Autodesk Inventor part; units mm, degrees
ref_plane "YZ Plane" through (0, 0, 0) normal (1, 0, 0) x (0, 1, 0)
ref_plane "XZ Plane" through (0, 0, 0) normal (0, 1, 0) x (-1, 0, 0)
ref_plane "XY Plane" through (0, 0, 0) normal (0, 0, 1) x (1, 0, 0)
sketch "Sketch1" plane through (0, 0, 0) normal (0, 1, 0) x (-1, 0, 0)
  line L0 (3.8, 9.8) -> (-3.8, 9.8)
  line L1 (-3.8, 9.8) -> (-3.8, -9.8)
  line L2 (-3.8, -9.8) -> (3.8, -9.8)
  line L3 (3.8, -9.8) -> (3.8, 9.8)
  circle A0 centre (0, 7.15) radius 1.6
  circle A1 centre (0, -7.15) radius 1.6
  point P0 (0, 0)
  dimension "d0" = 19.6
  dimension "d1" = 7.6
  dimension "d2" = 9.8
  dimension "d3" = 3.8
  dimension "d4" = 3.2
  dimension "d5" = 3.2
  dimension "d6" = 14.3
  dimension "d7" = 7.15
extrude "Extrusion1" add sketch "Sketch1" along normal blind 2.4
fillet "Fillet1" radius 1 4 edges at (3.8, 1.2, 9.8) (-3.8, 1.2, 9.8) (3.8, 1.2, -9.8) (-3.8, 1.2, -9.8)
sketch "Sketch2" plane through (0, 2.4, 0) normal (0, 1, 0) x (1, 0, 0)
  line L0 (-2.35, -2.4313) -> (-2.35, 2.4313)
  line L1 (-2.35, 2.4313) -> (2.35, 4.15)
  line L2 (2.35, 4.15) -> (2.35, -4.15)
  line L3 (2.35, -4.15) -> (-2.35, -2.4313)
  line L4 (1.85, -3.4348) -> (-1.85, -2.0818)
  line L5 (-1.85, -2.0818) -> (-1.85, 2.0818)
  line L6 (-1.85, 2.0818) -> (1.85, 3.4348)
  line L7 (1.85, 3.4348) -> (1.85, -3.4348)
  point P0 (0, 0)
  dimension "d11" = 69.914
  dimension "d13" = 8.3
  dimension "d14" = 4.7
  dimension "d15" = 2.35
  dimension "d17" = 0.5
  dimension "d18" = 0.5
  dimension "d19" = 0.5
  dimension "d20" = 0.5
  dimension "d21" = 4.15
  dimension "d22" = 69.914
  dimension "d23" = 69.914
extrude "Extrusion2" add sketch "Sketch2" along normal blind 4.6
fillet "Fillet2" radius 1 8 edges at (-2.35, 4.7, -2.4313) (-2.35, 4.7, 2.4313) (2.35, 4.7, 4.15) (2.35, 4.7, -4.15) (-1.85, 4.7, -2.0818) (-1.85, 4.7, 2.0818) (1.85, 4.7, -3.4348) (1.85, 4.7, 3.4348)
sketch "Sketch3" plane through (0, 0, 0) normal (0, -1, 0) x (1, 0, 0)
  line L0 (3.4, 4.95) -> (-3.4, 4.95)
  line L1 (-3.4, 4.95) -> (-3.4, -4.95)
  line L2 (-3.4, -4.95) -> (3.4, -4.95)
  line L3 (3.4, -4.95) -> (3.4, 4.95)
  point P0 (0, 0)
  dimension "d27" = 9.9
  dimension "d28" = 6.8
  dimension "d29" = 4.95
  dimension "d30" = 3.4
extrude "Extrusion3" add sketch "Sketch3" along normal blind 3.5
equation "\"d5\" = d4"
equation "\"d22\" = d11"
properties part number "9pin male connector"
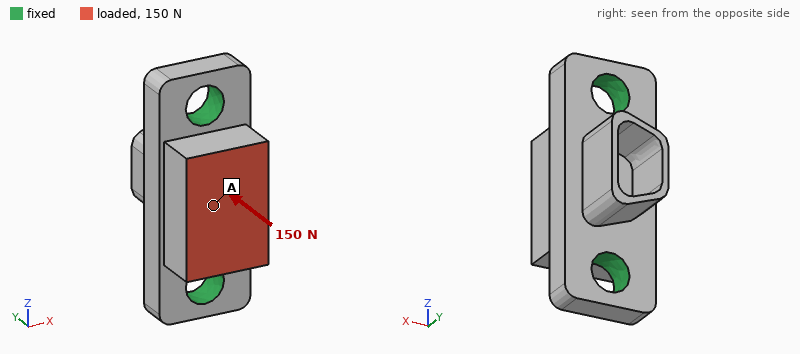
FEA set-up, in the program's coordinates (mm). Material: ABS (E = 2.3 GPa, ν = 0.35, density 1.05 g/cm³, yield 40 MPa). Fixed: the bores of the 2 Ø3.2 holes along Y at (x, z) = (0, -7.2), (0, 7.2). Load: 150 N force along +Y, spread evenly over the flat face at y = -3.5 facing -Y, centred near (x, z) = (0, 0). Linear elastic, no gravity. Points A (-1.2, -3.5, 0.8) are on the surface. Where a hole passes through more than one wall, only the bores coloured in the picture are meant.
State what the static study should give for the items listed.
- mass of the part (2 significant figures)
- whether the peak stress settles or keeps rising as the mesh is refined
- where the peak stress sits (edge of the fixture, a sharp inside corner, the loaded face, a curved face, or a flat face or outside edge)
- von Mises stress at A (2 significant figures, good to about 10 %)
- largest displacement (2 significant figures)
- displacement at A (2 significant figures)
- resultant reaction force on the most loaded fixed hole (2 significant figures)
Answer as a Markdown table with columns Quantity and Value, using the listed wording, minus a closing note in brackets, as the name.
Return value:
| Quantity | Value |
|---|---|
| mass of the part | 0.63 g |
| whether the peak stress settles or keeps rising as the mesh is refined | keeps rising |
| where the peak stress sits | edge of the fixture |
| von Mises stress at A | 3.0 MPa |
| largest displacement | 25 µm |
| displacement at A | 24 µm |
| resultant reaction force on the most loaded fixed hole | 81 N |
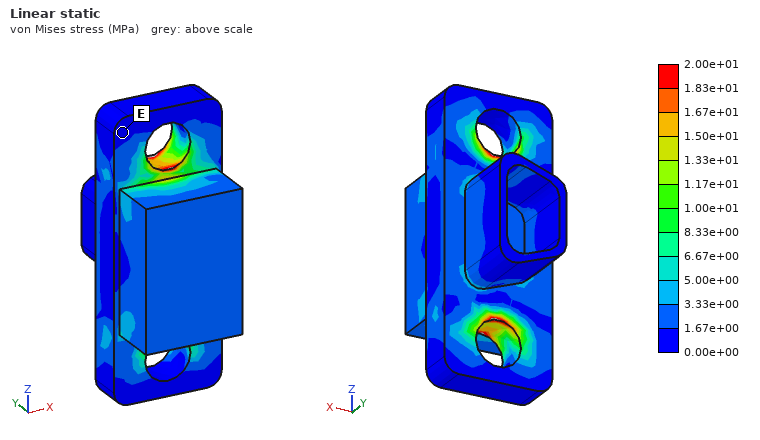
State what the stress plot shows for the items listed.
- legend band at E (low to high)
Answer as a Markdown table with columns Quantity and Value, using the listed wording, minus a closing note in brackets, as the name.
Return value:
| Quantity | Value |
|---|---|
| legend band at E | 0.00e+00 to 1.67e+00 MPa |
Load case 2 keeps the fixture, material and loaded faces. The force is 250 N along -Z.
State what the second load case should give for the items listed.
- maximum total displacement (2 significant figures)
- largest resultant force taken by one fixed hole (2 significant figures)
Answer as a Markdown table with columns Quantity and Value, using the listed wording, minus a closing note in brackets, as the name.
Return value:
| Quantity | Value |
|---|---|
| maximum total displacement | 56 µm |
| largest resultant force taken by one fixed hole | 160 N |
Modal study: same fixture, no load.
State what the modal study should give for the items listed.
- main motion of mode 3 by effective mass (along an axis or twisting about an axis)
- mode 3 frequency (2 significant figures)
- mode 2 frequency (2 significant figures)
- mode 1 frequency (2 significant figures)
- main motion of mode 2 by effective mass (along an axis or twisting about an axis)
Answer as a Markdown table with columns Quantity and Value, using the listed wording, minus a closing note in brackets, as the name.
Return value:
| Quantity | Value |
|---|---|
| main motion of mode 3 by effective mass | along Y |
| mode 3 frequency | 19 kHz |
| mode 2 frequency | 17 kHz |
| mode 1 frequency | 12 kHz |
| main motion of mode 2 by effective mass | along X |
